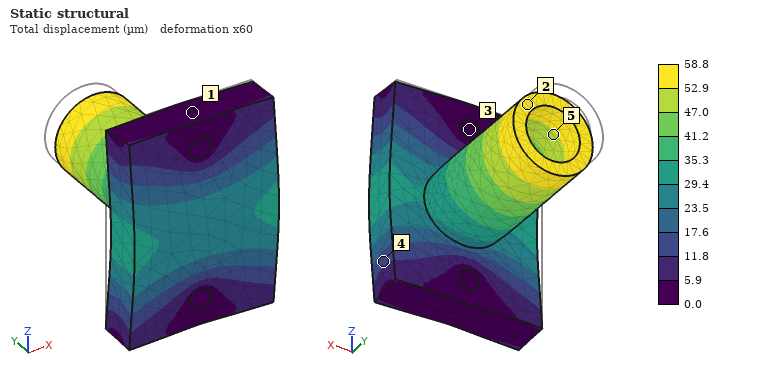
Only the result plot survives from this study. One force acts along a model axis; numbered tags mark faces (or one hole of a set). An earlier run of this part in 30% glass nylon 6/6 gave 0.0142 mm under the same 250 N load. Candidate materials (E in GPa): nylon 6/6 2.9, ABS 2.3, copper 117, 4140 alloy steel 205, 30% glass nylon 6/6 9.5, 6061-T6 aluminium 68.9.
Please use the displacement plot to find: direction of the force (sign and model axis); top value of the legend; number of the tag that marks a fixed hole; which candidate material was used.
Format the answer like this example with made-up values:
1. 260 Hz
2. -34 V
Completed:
1. -Y
2. 58.8 µm
3. 3
4. ABS
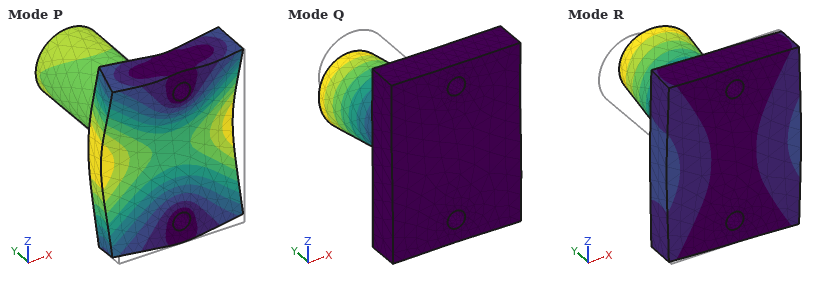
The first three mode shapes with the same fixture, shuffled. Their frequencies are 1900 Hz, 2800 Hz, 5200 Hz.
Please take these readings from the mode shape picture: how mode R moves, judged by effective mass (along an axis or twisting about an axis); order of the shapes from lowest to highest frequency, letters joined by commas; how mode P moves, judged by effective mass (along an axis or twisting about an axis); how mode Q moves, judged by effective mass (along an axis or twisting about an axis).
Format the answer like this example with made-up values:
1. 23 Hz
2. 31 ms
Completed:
1. along X
2. R, Q, P
3. along Y
4. along Z
